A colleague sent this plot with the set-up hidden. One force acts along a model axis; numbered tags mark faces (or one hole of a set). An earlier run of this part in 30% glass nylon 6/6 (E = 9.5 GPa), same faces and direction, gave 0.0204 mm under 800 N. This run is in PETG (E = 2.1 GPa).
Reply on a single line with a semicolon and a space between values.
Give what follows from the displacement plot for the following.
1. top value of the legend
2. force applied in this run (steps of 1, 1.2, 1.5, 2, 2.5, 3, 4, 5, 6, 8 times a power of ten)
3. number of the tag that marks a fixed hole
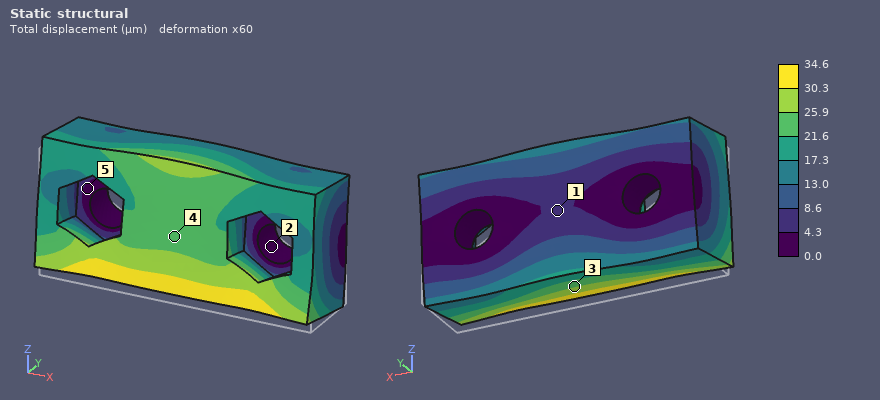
34.6 µm; 300 N; 2
